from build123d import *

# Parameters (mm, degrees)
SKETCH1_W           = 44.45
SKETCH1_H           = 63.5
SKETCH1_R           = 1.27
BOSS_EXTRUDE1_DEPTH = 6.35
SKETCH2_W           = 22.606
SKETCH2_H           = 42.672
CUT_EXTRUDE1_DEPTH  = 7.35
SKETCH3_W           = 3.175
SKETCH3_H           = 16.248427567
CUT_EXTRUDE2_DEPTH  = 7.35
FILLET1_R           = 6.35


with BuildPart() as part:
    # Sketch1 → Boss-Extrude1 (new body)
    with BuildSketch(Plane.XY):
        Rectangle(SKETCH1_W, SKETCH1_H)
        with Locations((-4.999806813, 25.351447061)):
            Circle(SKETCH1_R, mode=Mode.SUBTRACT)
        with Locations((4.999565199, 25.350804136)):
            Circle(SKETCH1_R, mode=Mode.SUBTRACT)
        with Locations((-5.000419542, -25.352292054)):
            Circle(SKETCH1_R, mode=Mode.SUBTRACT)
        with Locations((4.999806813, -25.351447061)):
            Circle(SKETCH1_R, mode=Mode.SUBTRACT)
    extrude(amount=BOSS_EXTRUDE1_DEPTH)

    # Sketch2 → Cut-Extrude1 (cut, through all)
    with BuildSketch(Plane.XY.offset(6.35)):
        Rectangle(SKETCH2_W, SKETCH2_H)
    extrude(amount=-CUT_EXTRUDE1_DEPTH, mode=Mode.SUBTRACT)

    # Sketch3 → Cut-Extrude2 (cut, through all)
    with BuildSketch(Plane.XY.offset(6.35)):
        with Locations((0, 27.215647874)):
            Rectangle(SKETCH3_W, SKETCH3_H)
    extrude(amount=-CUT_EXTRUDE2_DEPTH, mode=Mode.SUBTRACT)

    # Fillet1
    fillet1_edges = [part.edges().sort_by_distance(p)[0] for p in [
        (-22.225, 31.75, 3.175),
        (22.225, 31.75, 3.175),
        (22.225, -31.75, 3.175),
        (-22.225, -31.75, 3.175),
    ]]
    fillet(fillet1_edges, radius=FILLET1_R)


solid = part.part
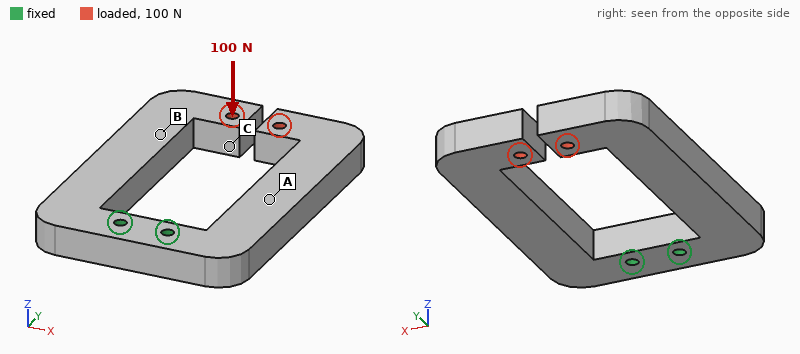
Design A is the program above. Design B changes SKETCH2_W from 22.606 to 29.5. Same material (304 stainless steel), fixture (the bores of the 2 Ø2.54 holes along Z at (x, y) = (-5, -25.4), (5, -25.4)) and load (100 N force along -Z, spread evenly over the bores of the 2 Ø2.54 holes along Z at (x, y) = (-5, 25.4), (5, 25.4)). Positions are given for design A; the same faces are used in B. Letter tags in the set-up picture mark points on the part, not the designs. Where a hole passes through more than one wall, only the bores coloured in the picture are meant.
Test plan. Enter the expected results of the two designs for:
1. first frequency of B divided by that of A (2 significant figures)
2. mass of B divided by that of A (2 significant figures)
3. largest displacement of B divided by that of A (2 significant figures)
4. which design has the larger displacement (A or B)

0.89
0.83
1.5
B
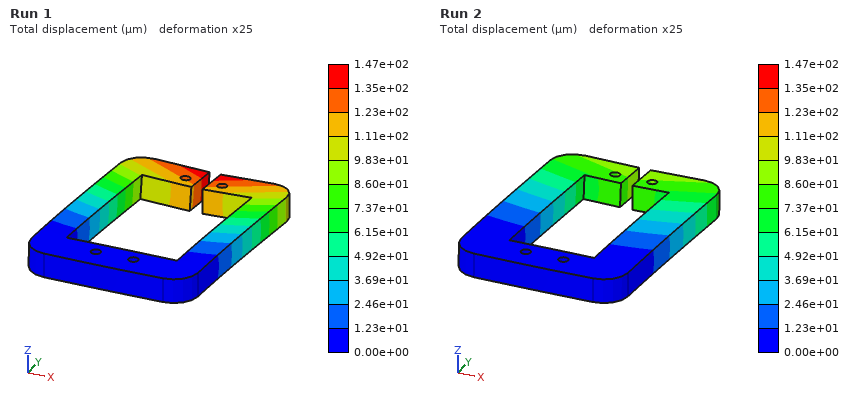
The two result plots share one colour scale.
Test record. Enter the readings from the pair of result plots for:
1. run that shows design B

Run 1
